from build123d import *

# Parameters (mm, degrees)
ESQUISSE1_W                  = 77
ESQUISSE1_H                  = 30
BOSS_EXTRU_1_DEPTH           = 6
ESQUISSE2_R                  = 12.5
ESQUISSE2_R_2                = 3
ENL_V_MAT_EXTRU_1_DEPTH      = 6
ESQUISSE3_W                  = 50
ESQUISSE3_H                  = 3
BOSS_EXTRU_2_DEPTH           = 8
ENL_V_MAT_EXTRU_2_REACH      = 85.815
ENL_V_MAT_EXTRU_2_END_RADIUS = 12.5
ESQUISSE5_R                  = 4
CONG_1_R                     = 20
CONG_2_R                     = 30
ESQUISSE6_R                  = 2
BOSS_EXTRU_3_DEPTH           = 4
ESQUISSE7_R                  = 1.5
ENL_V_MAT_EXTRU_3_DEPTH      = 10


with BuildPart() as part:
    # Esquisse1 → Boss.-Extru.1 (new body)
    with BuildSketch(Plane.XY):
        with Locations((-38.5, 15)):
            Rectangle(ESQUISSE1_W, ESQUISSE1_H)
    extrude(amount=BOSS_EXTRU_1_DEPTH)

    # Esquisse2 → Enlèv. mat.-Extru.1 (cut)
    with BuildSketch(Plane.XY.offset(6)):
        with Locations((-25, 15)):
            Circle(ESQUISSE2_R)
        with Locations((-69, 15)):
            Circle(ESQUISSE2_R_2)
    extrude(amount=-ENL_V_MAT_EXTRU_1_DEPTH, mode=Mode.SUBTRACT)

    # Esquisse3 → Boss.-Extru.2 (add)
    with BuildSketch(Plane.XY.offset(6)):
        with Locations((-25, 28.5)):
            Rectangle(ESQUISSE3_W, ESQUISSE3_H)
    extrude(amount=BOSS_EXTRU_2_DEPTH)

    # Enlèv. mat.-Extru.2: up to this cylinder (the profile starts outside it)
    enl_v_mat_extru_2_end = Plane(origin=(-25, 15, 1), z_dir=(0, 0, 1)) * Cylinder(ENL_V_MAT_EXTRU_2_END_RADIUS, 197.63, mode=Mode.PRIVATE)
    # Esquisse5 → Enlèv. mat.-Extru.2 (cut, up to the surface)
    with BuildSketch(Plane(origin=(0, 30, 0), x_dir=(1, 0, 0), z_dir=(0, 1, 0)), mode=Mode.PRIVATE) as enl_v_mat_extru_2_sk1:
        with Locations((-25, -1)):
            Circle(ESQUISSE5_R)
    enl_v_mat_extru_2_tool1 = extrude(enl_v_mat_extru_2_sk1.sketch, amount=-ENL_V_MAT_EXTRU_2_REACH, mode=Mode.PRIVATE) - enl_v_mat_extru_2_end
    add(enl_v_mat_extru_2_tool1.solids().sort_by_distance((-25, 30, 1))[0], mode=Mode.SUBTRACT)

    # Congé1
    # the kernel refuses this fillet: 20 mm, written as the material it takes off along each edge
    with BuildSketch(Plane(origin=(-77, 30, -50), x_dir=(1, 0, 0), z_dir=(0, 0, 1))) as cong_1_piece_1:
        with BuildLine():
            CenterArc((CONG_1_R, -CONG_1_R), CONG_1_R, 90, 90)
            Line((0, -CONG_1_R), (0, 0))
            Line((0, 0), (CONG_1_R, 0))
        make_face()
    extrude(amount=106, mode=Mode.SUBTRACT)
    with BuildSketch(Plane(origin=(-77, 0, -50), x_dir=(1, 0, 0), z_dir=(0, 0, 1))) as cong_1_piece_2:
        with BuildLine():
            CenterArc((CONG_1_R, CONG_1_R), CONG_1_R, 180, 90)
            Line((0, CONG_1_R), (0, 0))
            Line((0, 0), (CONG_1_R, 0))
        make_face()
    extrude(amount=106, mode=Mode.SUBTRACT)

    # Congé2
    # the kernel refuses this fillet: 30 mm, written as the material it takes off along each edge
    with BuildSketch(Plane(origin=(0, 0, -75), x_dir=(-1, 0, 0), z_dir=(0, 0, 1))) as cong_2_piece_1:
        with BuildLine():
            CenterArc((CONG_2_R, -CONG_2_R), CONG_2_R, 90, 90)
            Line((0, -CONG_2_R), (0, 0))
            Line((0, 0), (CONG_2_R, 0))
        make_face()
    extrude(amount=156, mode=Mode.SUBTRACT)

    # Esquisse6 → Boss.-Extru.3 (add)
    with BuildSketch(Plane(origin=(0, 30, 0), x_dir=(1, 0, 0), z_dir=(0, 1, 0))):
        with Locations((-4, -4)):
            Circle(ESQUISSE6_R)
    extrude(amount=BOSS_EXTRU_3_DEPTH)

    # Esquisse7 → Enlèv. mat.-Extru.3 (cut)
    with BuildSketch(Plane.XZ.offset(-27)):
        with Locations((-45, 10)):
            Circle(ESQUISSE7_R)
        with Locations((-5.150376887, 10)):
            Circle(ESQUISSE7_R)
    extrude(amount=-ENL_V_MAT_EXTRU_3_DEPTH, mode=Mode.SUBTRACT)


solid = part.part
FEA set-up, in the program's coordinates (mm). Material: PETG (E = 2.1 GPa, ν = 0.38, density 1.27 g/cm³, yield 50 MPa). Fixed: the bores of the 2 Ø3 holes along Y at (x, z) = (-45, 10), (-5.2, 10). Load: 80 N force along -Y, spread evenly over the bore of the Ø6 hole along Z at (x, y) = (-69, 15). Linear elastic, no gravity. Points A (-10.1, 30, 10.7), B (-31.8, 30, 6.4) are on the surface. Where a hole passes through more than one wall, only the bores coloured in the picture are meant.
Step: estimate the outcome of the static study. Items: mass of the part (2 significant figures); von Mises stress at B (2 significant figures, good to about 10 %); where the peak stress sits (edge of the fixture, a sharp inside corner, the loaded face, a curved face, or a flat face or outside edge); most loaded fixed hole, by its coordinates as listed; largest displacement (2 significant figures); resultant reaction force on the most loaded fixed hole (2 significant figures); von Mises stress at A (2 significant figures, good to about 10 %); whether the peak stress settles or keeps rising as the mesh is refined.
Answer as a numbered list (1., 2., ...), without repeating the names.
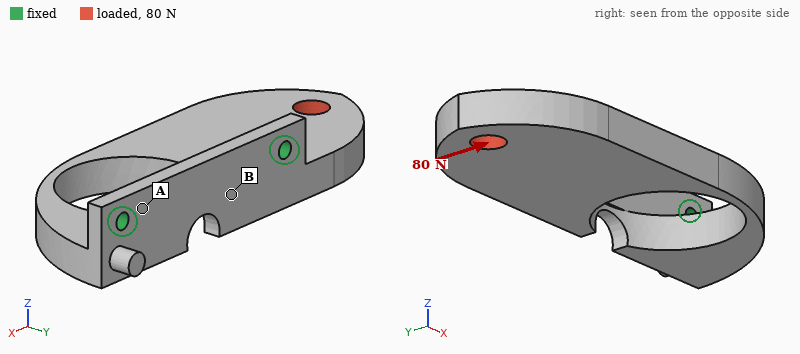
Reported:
1. 12 g
2. 7.4 MPa
3. edge of the fixture
4. (-45, 10)
5. 0.88 mm
6. 120 N
7. 3.7 MPa
8. keeps rising
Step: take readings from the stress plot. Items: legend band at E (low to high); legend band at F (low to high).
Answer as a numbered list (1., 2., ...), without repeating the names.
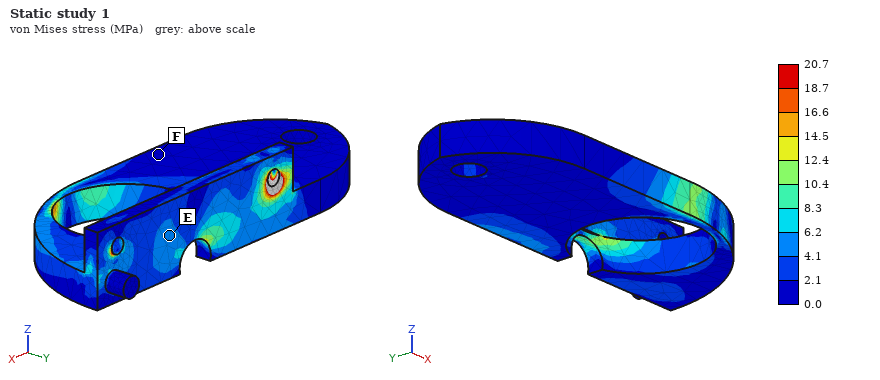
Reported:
1. 4.1 to 6.2 MPa
2. 0.0 to 2.1 MPa
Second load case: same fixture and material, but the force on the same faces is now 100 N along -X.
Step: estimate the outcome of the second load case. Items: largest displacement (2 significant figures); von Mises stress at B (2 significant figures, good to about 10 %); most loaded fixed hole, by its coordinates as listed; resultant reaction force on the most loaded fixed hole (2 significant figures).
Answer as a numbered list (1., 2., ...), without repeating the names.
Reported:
1. 0.26 mm
2. 3.4 MPa
3. (-45, 10)
4. 71 N
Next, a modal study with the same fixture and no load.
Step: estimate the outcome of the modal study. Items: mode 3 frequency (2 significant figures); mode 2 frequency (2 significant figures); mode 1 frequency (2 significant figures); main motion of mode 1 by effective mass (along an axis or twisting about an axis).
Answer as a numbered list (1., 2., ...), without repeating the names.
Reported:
1. 1100 Hz
2. 980 Hz
3. 410 Hz
4. along Z
